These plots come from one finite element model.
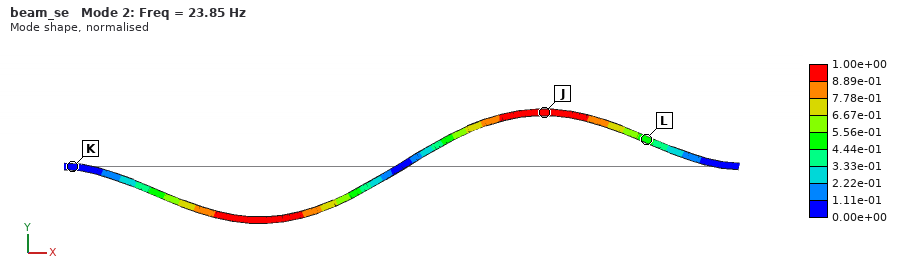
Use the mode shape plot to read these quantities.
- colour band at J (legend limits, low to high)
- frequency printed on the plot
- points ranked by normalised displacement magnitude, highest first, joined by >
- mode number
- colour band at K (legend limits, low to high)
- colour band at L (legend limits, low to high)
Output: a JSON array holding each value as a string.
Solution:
["8.89e-01 to 1.00e+00", "23.85 Hz", "J > L > K", "2", "0.00e+00 to 1.11e-01", "4.44e-01 to 5.56e-01"]
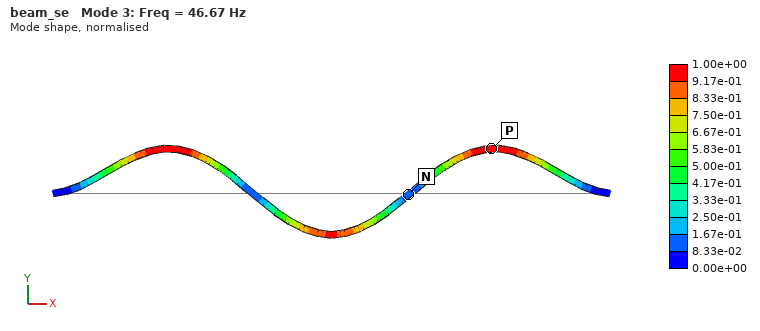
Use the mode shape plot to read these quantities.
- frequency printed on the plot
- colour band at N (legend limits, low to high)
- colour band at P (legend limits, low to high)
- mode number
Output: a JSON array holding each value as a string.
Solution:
["46.67 Hz", "8.33e-02 to 1.67e-01", "9.17e-01 to 1.00e+00", "3"]
